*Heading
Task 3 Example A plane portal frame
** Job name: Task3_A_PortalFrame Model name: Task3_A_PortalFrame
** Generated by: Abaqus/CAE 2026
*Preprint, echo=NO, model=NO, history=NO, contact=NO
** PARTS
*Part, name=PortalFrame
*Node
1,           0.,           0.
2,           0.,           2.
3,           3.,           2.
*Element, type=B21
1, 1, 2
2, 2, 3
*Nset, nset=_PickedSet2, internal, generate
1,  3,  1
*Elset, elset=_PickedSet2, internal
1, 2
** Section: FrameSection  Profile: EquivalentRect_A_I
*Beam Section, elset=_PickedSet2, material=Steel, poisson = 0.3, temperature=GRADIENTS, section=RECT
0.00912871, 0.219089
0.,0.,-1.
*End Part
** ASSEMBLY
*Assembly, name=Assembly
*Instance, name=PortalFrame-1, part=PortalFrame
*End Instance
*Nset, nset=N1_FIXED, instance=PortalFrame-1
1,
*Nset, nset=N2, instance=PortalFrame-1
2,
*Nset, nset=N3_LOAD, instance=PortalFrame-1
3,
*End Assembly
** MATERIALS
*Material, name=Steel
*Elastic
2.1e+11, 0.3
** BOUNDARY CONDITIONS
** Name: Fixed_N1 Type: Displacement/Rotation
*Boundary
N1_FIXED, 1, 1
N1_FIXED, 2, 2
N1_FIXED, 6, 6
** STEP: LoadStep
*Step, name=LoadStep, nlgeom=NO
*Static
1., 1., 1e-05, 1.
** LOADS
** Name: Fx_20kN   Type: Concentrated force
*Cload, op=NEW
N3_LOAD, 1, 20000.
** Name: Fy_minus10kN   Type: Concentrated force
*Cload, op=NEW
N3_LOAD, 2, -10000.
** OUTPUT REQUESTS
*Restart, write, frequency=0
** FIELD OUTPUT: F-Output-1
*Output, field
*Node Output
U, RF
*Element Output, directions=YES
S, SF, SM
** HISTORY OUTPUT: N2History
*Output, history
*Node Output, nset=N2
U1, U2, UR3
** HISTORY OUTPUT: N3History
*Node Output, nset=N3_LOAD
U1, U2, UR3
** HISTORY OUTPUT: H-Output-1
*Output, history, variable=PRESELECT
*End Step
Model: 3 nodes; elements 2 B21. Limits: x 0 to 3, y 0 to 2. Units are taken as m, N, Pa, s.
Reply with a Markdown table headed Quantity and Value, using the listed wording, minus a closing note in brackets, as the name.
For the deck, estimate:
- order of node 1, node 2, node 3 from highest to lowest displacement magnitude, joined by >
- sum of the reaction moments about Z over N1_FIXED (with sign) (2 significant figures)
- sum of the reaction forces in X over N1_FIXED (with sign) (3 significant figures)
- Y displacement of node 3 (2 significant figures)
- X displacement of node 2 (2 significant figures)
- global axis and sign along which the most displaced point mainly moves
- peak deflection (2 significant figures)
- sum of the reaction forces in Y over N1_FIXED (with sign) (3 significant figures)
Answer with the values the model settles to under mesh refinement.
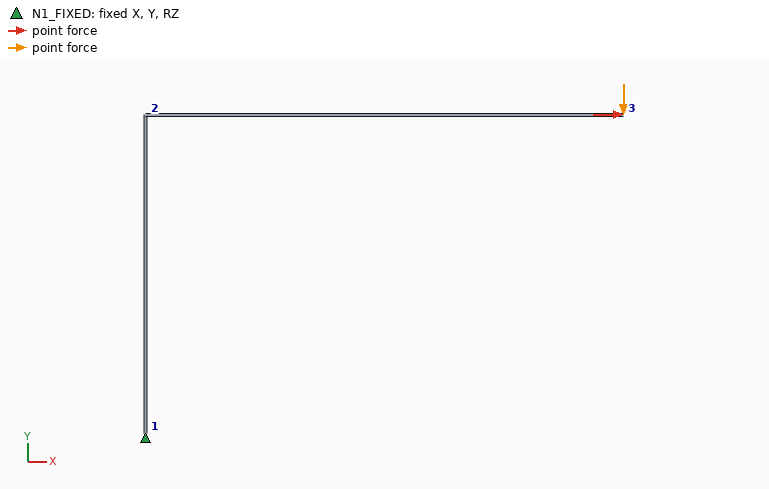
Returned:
| Quantity | Value |
|---|---|
| order of node 1, node 2, node 3 from highest to lowest displacement magnitude, joined by > | node 3 > node 2 > node 1 |
| sum of the reaction moments about Z over N1_FIXED (with sign) | 70000 N·m |
| sum of the reaction forces in X over N1_FIXED (with sign) | -20000 N |
| Y displacement of node 3 | -0.23 m |
| X displacement of node 2 | 0.068 m |
| global axis and sign along which the most displaced point mainly moves | -Y |
| peak deflection | 0.24 m |
| sum of the reaction forces in Y over N1_FIXED (with sign) | 10000 N |
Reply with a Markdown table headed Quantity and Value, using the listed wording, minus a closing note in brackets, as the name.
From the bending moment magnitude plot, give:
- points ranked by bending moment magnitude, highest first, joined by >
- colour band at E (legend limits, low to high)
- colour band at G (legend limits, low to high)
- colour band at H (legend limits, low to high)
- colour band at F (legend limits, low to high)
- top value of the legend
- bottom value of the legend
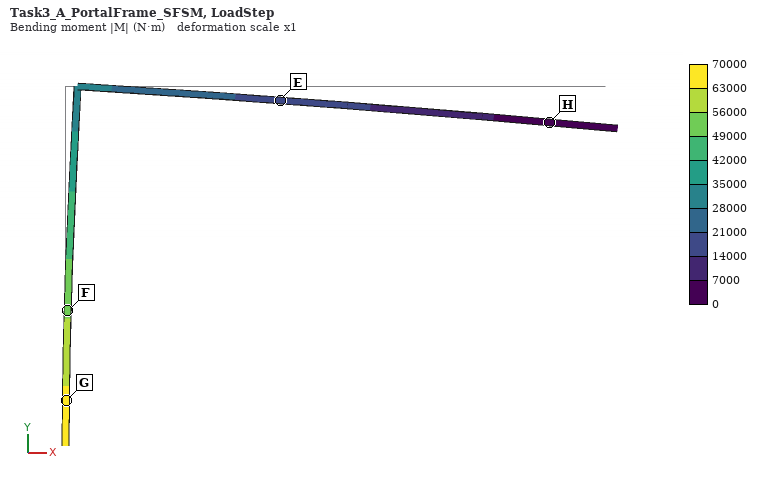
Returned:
| Quantity | Value |
|---|---|
| points ranked by bending moment magnitude, highest first, joined by > | G > F > E > H |
| colour band at E | 14000 to 21000 N·m |
| colour band at G | 63000 to 70000 N·m |
| colour band at H | 0 to 7000 N·m |
| colour band at F | 49000 to 56000 N·m |
| top value of the legend | 70000 N·m |
| bottom value of the legend | 0 N·m |
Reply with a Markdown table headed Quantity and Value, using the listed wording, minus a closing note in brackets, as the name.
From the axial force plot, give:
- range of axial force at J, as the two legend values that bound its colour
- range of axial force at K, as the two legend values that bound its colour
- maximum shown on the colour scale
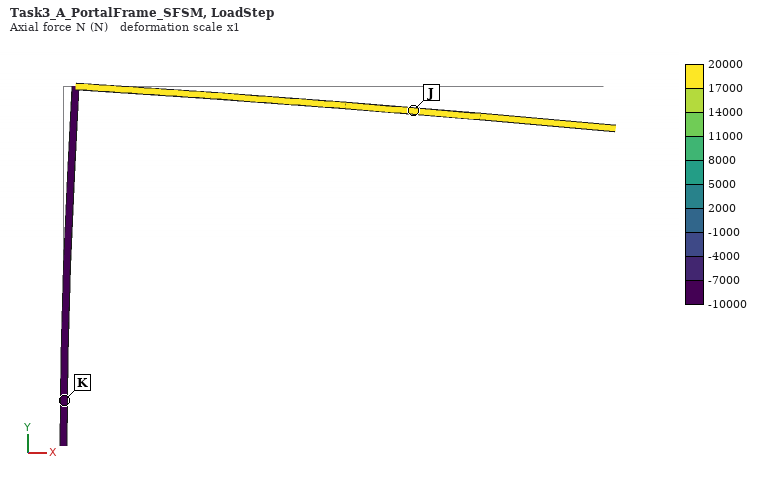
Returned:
| Quantity | Value |
|---|---|
| range of axial force at J, as the two legend values that bound its colour | 17000 to 20000 N |
| range of axial force at K, as the two legend values that bound its colour | -10000 to -7000 N |
| maximum shown on the colour scale | 20000 N |
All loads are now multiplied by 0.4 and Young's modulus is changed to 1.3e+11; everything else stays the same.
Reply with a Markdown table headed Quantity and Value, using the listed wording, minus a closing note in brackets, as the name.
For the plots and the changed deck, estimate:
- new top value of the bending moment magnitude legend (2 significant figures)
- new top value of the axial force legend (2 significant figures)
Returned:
| Quantity | Value |
|---|---|
| new top value of the bending moment magnitude legend | 28000 N·m |
| new top value of the axial force legend | 8000 N |
